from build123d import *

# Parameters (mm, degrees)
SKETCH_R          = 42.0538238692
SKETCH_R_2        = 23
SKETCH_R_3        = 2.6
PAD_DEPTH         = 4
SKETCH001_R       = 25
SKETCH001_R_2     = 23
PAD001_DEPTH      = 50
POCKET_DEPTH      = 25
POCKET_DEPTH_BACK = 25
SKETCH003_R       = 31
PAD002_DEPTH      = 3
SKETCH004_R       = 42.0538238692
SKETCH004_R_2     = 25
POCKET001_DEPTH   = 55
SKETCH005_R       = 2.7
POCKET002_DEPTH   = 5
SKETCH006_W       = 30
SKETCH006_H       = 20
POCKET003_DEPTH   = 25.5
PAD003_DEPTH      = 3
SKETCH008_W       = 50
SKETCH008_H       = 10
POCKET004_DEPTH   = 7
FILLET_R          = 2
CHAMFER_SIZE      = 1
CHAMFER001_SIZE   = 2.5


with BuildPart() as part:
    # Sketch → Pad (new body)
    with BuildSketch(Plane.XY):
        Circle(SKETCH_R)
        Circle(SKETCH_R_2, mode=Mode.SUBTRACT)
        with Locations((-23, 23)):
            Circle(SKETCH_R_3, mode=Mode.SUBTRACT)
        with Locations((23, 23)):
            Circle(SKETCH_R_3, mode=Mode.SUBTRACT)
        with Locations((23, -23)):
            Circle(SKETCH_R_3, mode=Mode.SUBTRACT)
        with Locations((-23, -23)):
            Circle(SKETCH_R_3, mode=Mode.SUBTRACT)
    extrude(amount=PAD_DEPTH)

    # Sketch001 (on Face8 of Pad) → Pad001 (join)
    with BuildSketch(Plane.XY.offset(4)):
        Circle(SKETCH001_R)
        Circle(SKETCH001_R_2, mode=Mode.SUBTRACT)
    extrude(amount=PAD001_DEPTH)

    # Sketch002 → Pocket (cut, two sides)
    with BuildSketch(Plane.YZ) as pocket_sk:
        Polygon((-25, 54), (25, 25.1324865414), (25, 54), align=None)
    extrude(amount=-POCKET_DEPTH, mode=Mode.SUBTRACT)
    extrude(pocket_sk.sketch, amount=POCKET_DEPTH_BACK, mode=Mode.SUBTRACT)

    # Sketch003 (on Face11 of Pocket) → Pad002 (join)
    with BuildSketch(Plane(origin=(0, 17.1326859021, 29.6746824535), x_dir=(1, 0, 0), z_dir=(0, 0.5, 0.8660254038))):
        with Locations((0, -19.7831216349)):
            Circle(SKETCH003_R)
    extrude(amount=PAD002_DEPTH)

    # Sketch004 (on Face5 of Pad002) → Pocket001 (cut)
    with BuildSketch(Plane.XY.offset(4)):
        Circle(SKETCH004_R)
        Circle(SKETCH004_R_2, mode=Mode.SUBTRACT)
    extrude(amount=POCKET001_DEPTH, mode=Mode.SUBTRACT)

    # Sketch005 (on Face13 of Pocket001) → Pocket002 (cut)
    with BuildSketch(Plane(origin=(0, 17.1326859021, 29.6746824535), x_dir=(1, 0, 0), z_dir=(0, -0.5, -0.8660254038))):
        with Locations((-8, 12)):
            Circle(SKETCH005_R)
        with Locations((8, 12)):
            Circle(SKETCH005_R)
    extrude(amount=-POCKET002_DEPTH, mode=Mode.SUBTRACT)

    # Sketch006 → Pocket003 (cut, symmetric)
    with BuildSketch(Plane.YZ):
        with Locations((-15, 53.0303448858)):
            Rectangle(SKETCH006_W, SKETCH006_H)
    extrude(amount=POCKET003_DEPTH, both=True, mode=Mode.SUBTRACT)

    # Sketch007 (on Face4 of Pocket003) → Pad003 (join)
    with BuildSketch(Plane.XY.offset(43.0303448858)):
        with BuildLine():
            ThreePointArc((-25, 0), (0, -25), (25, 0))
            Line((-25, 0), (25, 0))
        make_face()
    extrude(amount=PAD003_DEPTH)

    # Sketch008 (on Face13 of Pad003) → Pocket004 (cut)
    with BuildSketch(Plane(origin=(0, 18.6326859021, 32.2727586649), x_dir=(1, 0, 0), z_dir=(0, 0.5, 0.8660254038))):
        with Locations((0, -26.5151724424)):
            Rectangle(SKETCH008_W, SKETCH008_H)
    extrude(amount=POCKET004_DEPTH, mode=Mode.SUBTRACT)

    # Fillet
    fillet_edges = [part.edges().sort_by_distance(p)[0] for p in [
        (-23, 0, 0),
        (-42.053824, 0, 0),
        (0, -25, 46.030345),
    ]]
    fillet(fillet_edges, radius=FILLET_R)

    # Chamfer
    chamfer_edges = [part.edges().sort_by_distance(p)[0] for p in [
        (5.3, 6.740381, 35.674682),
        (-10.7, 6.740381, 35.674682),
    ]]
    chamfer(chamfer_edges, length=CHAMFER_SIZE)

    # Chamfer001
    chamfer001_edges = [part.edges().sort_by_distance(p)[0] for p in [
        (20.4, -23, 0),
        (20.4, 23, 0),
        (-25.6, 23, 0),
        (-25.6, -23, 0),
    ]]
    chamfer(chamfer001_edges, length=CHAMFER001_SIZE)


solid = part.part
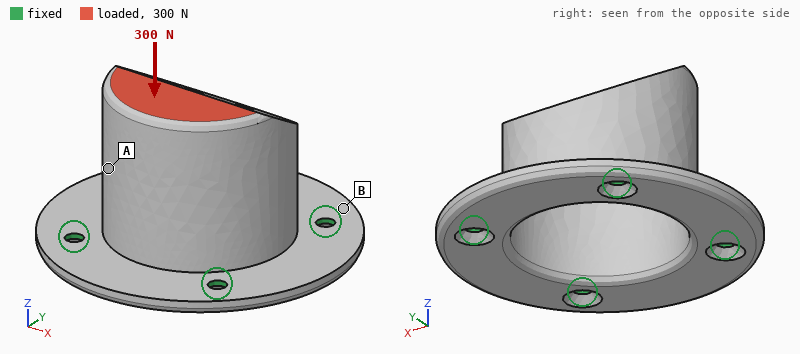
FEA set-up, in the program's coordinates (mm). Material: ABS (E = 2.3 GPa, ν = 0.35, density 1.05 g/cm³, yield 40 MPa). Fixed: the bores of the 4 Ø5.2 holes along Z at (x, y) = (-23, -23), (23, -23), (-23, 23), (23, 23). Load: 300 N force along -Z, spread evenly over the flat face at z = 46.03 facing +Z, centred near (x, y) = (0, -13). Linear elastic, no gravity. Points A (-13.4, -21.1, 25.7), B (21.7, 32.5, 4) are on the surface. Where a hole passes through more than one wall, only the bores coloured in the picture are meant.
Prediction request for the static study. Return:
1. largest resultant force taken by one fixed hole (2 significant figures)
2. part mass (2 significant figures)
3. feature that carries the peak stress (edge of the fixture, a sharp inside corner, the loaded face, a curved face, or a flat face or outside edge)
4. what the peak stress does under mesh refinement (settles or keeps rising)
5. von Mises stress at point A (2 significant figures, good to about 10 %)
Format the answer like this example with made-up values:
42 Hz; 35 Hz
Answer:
120 N; 32 g; edge of the fixture; keeps rising; 2.4 MPa
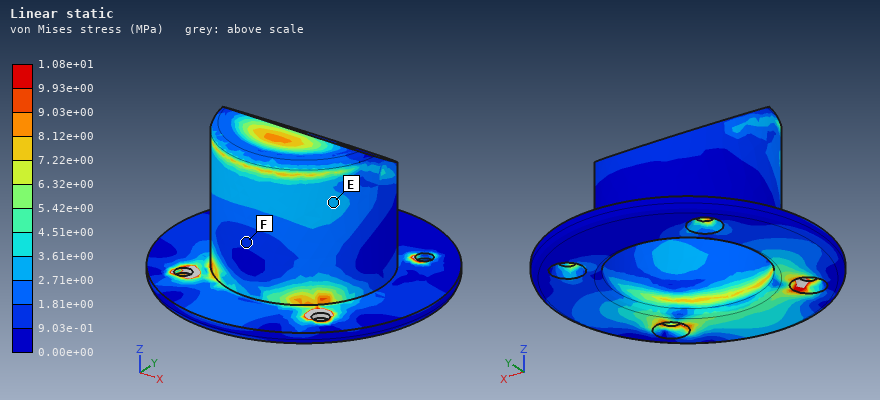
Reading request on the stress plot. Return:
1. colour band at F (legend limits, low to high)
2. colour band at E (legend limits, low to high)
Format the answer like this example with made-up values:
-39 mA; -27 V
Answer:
9.03e-01 to 1.81e+00 MPa; 2.71e+00 to 3.61e+00 MPa
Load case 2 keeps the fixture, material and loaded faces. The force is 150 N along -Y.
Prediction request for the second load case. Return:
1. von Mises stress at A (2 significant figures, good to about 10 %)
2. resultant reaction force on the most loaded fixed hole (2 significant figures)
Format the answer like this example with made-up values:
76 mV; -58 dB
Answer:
1.1 MPa; 93 N
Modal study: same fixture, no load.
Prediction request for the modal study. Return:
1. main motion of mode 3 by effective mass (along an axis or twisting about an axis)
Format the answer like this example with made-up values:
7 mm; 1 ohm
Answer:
along Z
